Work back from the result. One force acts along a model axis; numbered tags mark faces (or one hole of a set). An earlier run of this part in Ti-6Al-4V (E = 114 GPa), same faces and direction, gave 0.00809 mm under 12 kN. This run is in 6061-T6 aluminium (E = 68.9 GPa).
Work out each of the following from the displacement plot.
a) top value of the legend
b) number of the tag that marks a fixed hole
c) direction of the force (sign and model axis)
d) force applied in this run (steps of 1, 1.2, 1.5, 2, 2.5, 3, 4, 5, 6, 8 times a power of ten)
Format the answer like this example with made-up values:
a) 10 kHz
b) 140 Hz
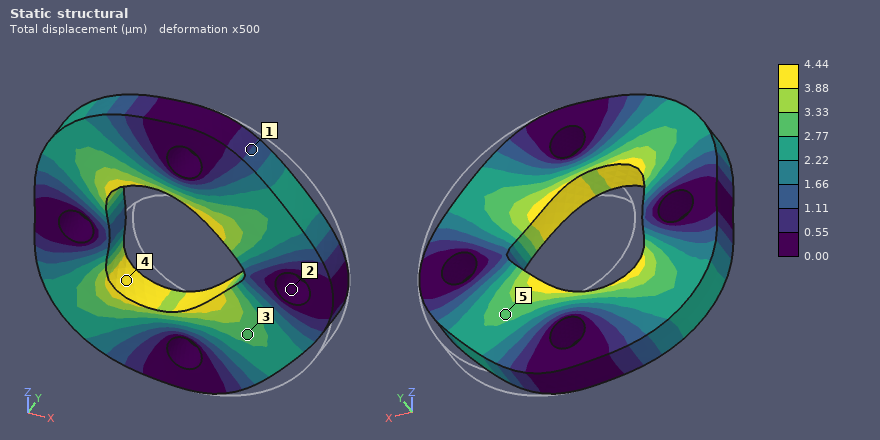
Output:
a) 4.44 µm
b) 2
c) -X
d) 4 kN
